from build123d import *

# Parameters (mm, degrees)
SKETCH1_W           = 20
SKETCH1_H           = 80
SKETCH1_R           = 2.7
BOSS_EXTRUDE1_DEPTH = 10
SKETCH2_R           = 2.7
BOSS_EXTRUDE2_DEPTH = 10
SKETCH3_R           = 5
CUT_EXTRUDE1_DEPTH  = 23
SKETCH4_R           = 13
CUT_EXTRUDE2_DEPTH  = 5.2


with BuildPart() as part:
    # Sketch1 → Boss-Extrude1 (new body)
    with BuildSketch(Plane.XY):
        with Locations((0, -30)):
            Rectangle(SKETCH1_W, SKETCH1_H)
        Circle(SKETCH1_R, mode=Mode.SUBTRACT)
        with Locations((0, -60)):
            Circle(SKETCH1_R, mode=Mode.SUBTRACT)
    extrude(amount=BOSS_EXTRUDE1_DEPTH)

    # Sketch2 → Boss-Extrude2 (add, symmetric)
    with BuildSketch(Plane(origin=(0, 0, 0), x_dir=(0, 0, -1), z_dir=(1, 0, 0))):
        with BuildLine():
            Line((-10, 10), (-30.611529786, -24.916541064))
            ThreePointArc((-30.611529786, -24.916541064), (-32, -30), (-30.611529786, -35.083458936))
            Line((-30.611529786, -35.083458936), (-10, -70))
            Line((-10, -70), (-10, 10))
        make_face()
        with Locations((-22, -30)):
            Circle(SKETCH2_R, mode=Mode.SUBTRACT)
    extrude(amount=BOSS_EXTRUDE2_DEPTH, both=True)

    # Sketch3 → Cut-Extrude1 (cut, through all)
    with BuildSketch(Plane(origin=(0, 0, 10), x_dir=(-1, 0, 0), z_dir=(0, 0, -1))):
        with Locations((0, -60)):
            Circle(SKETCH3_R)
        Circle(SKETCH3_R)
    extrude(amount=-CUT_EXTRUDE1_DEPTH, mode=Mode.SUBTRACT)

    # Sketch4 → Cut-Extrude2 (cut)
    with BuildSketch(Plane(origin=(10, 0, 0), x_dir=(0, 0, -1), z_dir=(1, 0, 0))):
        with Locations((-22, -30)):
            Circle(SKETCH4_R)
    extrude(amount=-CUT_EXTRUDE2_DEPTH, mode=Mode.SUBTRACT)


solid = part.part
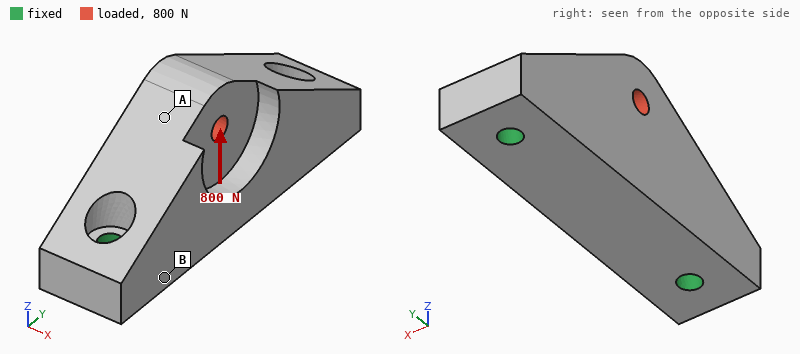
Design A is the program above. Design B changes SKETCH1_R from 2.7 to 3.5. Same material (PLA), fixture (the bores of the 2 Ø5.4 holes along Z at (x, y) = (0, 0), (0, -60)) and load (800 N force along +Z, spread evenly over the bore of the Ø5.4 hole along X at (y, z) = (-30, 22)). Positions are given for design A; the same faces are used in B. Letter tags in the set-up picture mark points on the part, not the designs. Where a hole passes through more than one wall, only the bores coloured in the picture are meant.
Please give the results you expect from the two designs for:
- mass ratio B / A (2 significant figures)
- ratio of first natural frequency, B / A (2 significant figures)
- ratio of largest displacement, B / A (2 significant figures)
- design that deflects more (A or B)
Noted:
0.99
1.1
0.87
A
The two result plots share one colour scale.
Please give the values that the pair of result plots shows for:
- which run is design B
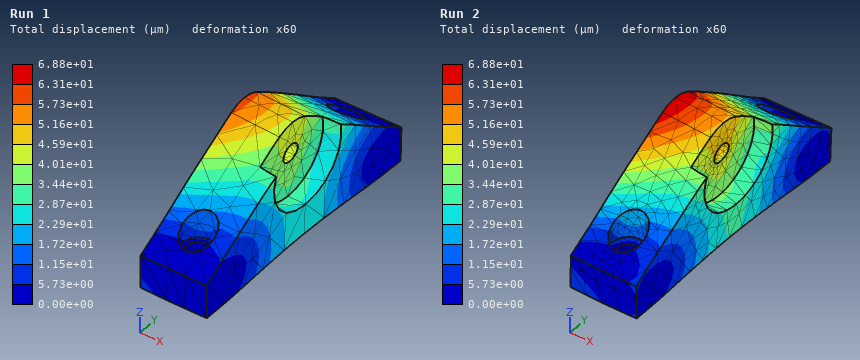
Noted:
Run 1
